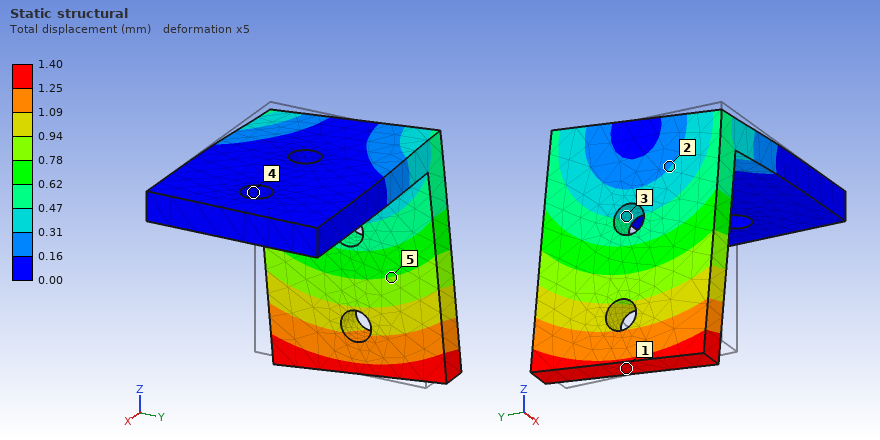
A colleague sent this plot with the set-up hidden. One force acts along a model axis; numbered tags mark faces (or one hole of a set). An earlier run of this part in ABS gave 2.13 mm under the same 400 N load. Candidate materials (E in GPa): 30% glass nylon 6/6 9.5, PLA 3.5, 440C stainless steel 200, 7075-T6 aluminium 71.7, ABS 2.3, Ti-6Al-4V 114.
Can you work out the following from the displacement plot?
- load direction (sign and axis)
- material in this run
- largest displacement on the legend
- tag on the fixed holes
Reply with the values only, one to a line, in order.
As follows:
+Y
PLA
1.40 mm
4
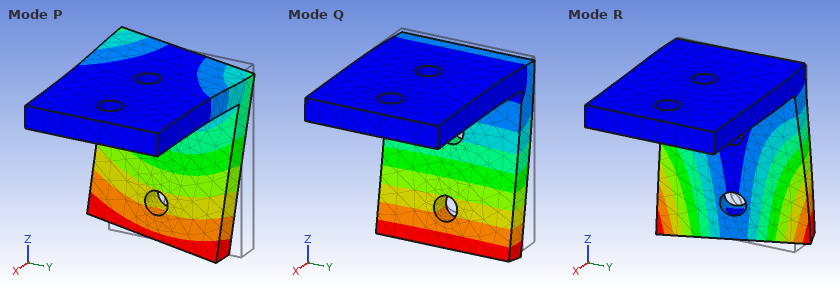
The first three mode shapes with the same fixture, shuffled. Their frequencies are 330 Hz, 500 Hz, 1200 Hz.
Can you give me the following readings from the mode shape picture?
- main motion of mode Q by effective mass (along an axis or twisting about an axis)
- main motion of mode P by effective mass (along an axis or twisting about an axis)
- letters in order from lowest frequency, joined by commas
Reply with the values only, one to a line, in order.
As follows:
along X
along Y
Q, P, R
